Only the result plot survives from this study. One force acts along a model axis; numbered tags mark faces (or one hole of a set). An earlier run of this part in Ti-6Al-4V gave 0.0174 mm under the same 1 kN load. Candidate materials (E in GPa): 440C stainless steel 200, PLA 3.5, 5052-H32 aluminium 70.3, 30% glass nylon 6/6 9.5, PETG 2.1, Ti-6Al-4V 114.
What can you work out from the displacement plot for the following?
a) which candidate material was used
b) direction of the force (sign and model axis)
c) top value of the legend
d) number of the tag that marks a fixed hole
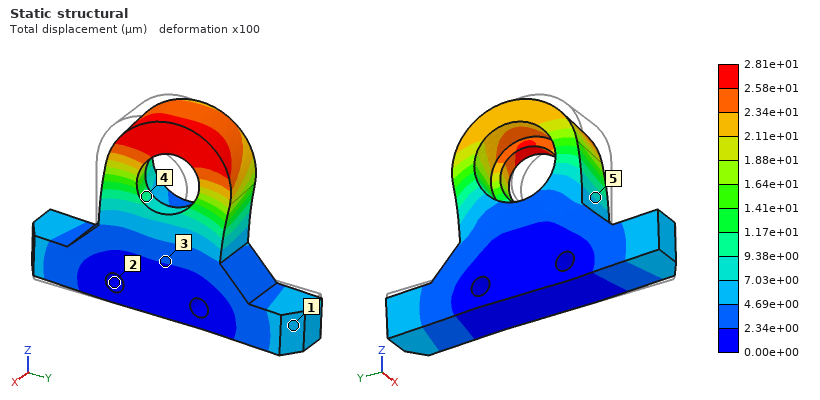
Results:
5052-H32 aluminium
+Y
2.81e+01 µm
2
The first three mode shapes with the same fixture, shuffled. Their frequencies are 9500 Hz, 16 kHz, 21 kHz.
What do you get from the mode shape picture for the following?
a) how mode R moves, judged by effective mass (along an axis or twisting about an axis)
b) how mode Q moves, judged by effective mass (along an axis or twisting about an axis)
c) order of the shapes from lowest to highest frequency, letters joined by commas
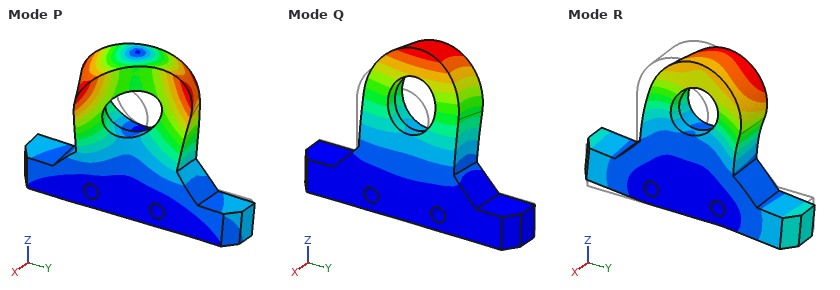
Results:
along Y
along X
Q, R, P
